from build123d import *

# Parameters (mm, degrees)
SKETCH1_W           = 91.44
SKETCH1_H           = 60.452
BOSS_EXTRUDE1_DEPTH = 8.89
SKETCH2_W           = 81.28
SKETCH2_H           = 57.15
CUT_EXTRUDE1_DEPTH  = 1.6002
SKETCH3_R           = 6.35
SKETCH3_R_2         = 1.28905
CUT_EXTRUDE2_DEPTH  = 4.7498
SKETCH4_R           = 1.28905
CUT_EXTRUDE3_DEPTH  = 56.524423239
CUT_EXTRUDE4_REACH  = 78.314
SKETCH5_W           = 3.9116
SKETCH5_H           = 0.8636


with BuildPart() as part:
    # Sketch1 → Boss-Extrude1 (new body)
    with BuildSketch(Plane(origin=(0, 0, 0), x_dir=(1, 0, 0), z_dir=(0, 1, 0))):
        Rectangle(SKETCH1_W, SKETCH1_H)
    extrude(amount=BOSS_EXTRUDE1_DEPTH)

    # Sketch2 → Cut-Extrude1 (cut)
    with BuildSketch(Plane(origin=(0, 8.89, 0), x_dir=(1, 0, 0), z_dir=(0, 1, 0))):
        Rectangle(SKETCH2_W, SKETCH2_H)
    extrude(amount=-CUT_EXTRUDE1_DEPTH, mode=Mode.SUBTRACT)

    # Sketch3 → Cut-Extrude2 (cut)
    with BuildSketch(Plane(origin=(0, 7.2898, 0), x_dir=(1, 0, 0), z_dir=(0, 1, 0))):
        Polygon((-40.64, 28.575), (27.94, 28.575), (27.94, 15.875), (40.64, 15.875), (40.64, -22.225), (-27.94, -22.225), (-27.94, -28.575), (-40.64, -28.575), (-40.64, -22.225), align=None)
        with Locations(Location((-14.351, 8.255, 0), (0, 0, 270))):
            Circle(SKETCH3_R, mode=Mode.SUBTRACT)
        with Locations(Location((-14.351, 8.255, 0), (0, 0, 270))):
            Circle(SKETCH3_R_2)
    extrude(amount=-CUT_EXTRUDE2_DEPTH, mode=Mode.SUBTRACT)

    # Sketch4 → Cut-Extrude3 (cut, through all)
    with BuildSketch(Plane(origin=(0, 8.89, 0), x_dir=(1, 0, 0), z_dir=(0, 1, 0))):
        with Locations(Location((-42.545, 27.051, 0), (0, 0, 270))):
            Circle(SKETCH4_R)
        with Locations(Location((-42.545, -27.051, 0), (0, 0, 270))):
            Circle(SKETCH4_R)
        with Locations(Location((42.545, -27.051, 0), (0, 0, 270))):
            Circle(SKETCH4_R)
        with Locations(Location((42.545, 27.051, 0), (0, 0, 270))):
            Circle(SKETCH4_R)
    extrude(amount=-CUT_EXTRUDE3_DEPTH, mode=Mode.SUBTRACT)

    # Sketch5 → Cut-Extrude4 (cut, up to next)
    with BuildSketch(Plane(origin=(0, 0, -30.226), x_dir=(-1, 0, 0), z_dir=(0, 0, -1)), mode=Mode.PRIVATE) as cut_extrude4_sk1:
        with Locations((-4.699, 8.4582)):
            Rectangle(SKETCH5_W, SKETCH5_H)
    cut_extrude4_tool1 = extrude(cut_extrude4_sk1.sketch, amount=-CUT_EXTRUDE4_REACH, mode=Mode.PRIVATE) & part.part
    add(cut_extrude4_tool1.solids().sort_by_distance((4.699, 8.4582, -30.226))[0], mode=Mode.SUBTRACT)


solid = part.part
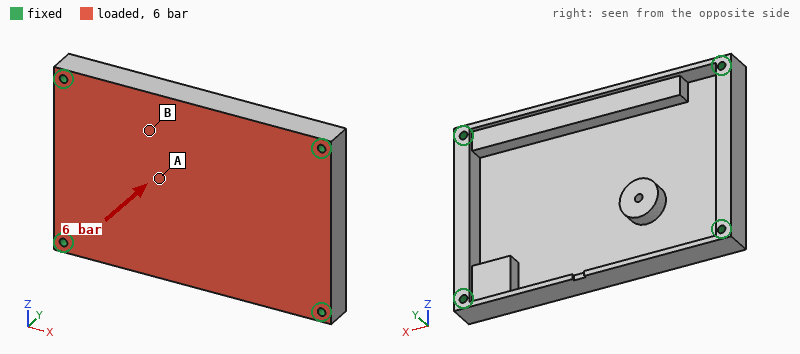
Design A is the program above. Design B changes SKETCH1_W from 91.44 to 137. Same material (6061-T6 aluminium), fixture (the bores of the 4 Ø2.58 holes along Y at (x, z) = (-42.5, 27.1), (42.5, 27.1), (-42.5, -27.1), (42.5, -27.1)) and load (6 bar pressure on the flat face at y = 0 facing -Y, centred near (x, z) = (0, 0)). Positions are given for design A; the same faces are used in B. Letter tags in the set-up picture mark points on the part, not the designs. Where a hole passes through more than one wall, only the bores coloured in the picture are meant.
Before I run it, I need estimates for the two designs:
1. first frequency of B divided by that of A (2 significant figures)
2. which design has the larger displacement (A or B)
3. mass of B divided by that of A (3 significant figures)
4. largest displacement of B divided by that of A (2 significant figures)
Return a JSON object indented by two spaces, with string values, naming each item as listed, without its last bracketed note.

{
  "first frequency of B divided by that of A": "1.0",
  "which design has the larger displacement": "A",
  "mass of B divided by that of A": "2.07",
  "largest displacement of B divided by that of A": "0.90"
}
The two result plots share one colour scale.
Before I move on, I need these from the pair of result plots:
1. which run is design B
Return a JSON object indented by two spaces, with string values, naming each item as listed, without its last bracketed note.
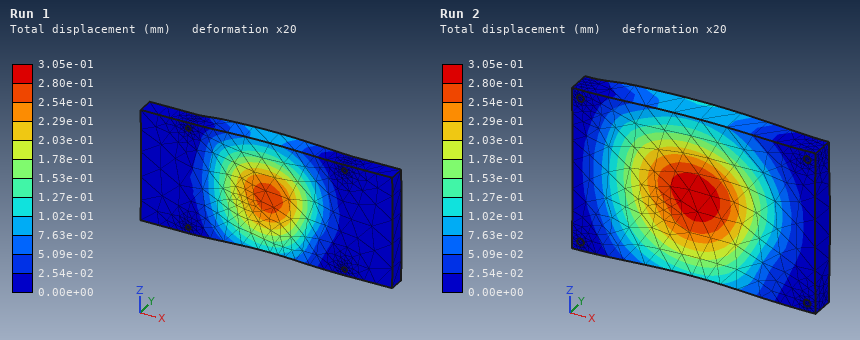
{
  "which run is design B": "Run 1"
}
